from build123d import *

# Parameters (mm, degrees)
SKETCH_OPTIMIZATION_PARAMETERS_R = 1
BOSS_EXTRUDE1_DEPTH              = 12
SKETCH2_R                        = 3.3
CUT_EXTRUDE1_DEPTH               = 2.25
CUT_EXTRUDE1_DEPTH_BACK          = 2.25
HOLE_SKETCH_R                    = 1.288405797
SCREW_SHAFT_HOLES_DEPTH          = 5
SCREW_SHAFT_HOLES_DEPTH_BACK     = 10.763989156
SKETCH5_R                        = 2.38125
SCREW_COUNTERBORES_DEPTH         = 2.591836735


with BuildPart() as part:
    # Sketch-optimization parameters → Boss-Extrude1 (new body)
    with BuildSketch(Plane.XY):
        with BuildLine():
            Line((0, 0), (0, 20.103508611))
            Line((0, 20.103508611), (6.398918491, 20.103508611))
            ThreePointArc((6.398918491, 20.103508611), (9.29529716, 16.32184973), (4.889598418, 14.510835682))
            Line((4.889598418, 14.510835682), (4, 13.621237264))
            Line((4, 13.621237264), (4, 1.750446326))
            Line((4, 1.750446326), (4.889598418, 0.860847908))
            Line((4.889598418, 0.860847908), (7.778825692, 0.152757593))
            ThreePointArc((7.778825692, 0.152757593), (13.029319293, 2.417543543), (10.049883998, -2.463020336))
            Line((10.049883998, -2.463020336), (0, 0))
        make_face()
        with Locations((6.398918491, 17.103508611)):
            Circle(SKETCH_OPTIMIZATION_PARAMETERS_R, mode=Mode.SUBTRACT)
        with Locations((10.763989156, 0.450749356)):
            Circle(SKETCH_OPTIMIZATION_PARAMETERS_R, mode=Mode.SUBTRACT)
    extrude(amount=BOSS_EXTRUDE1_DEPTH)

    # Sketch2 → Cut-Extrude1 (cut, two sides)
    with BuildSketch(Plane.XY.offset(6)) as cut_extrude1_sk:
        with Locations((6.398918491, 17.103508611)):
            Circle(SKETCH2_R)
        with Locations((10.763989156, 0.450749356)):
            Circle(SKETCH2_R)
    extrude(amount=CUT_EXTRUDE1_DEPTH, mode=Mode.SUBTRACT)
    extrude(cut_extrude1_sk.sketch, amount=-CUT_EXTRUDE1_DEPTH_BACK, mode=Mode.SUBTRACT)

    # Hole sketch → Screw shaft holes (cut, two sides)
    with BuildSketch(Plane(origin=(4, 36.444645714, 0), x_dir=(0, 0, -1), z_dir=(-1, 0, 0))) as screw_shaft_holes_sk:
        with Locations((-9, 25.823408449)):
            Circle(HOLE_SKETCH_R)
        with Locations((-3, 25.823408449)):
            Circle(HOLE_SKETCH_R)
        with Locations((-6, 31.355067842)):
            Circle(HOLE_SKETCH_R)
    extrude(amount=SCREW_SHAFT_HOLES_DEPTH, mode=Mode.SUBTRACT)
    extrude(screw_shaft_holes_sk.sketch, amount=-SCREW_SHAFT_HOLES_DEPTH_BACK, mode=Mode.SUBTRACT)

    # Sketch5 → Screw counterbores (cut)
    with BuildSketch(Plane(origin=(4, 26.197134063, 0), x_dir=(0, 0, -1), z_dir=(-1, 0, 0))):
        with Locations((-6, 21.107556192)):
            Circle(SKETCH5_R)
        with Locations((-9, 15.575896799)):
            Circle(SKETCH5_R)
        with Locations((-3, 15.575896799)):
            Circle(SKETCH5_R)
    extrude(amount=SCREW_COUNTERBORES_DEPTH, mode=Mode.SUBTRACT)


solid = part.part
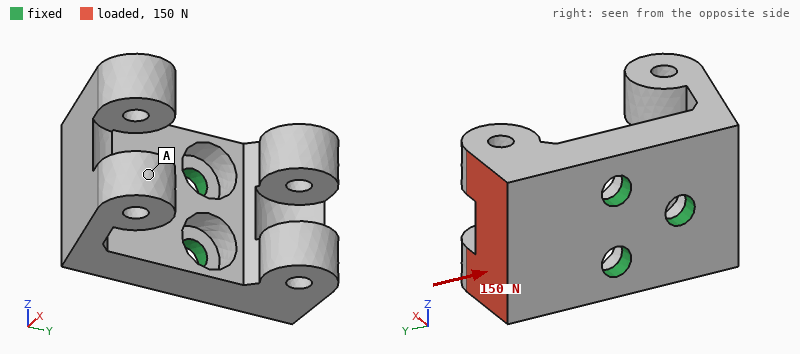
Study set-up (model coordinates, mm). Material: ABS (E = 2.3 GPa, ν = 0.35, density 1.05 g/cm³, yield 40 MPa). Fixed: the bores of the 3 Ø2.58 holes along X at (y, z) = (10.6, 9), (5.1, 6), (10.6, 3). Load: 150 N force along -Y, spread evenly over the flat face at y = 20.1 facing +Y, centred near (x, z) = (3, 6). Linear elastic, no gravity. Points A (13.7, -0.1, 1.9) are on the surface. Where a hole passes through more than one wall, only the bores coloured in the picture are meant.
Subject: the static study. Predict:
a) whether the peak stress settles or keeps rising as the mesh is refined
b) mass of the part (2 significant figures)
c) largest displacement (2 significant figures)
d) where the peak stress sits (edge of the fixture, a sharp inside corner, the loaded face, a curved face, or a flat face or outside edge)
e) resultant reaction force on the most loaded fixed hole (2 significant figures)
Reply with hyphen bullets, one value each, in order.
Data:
- keeps rising
- 1.4 g
- 0.22 mm
- a sharp inside corner
- 59 N
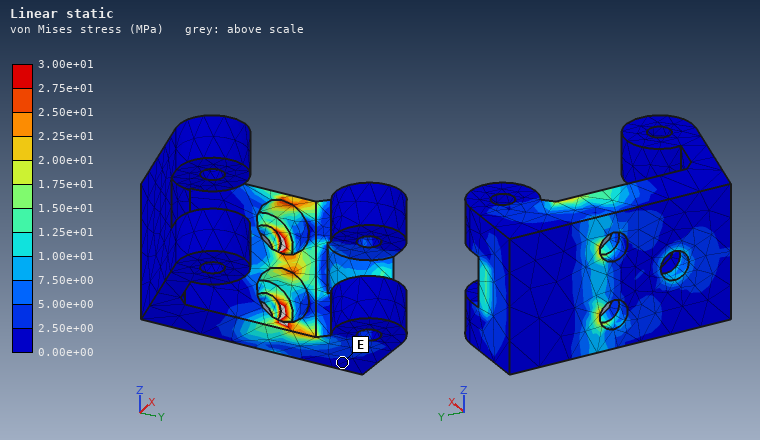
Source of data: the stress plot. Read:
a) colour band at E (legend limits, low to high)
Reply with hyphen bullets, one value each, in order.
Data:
- 0.00e+00 to 2.50e+00 MPa
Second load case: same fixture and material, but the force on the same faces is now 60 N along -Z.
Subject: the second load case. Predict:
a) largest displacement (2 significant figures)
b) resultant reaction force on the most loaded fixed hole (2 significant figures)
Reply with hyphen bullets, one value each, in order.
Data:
- 66 µm
- 73 N
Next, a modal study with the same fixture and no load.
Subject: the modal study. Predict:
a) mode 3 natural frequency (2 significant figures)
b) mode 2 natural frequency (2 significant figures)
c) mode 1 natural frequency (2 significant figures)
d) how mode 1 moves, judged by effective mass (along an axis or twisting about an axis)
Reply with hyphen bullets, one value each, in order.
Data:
- 4000 Hz
- 3200 Hz
- 2800 Hz
- along Y
